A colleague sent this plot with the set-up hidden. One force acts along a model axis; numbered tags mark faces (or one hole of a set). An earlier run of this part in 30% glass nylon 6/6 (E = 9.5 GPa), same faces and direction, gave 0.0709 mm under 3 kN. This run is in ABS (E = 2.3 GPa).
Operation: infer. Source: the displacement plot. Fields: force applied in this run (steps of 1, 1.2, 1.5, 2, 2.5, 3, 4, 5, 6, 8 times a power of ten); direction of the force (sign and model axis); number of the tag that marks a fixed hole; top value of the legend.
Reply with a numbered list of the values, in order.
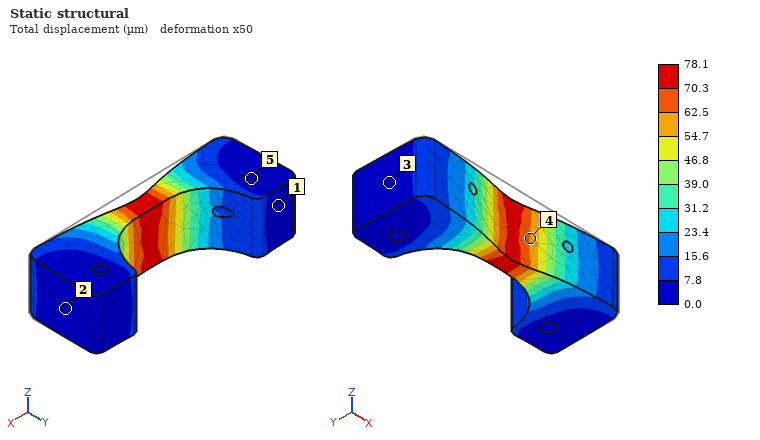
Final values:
1. 800 N
2. +Y
3. 5
4. 78.1 µm
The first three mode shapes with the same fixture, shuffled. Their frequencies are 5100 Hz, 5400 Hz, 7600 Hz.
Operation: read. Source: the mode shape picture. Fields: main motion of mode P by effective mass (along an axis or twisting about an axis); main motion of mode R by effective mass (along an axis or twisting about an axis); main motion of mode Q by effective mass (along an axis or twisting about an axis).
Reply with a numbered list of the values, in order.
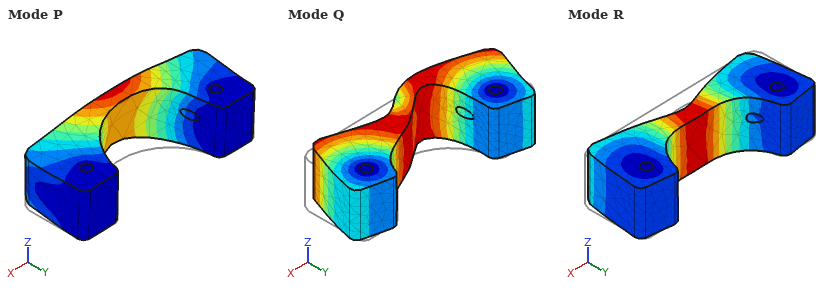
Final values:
1. along Z
2. along Y
3. along X
